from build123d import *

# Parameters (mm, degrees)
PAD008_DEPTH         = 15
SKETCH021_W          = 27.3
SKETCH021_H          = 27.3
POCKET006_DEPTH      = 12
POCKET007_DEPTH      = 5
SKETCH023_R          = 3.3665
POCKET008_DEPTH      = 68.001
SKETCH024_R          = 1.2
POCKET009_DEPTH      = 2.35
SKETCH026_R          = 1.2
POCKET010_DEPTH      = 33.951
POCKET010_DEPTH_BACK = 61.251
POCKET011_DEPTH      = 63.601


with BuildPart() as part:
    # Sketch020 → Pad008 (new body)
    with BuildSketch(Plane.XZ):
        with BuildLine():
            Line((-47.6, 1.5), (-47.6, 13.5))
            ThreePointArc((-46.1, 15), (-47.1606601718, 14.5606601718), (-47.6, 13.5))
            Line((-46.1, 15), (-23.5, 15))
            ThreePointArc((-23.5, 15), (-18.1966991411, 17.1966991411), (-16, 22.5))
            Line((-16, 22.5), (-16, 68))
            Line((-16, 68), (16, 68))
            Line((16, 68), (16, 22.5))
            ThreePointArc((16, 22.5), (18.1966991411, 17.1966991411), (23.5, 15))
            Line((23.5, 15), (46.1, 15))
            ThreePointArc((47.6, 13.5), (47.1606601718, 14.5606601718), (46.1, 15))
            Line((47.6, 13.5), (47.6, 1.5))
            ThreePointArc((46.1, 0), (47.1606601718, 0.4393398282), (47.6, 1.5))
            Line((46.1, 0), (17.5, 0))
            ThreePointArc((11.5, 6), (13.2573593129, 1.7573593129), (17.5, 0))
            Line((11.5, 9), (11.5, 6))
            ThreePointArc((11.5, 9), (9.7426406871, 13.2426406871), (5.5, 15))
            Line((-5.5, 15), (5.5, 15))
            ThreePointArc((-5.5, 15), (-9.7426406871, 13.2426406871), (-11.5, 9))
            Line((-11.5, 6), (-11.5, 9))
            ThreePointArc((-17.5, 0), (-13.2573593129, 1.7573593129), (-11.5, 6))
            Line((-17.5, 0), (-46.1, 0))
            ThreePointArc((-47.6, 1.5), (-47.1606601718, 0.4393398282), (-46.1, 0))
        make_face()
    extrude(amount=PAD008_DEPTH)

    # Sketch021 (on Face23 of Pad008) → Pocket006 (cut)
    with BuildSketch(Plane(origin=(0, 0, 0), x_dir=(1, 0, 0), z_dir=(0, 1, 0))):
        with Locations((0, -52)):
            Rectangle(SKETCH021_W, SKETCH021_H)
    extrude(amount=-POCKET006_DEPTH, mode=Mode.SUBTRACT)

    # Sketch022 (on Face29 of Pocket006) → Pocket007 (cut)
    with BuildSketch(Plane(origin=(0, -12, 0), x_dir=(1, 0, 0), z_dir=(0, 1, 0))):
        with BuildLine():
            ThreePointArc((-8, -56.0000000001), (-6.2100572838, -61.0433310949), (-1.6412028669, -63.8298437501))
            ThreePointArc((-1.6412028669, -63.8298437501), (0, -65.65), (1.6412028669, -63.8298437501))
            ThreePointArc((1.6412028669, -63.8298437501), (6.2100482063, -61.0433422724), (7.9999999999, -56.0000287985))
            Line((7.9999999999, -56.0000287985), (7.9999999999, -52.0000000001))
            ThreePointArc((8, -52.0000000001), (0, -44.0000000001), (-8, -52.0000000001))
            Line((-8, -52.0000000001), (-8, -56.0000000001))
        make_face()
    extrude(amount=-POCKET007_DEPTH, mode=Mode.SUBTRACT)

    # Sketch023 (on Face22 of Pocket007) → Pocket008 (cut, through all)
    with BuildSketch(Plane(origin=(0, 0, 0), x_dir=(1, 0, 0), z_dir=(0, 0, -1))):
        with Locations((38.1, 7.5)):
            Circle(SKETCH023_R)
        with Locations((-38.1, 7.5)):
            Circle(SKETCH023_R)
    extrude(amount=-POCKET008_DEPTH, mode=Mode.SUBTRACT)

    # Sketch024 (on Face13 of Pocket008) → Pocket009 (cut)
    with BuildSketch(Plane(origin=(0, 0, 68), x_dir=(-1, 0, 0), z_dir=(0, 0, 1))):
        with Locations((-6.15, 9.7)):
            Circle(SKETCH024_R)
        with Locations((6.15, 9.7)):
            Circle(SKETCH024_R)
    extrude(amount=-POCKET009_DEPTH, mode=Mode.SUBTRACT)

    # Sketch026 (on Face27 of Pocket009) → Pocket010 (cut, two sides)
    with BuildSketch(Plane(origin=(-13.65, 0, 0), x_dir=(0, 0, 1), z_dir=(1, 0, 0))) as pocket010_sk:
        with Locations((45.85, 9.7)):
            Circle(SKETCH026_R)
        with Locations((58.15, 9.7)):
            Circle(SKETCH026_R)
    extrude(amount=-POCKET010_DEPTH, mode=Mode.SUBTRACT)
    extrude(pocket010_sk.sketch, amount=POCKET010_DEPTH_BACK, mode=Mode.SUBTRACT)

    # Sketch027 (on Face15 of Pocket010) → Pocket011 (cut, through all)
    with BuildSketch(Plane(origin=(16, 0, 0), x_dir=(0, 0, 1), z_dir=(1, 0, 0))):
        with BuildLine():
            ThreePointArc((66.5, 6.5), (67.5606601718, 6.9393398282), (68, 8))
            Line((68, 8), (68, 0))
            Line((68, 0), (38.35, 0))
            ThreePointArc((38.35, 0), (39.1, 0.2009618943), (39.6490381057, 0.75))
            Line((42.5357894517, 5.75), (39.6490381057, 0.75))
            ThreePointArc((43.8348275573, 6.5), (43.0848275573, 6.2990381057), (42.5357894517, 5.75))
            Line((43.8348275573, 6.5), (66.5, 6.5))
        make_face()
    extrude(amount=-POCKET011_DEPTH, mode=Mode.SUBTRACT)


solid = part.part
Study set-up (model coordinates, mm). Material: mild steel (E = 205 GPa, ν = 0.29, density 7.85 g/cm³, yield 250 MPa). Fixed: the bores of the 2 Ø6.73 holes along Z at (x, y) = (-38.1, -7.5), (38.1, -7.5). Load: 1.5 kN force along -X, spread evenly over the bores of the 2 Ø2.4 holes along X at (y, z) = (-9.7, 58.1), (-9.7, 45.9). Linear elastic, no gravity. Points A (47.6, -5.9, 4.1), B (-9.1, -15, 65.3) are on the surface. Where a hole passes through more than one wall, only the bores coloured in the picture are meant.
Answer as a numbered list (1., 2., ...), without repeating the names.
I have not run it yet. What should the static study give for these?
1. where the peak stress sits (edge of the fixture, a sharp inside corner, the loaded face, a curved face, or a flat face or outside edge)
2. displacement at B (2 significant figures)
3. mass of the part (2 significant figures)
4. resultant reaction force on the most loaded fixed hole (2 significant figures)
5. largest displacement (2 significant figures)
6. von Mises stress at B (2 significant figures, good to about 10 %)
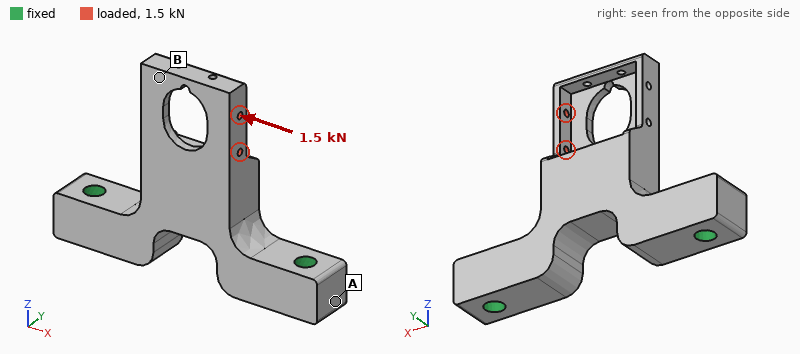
1. the loaded face
2. 40 µm
3. 230 g
4. 1.6 kN
5. 66 µm
6. 33 MPa
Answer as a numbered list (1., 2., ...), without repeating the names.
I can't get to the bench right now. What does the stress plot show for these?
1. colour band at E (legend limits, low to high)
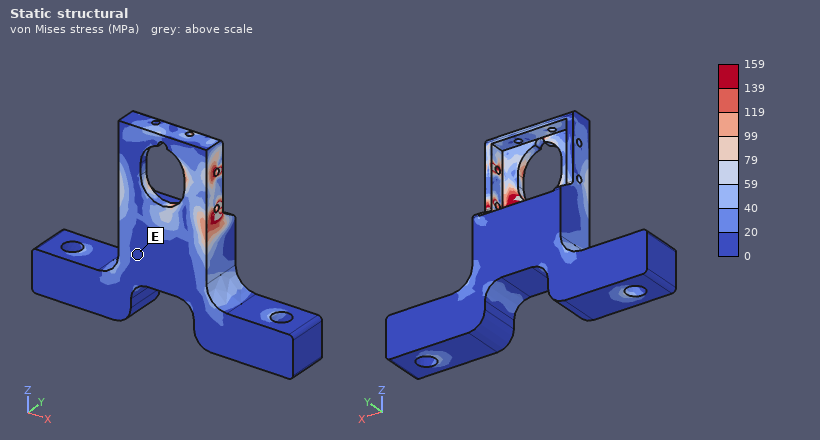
1. 0 to 20 MPa
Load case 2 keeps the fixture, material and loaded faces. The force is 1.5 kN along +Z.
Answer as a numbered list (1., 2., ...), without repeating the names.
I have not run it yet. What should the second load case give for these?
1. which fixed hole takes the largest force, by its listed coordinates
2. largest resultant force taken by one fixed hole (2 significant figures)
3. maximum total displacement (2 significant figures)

1. (38.1, -7.5)
2. 1.4 kN
3. 21 µm
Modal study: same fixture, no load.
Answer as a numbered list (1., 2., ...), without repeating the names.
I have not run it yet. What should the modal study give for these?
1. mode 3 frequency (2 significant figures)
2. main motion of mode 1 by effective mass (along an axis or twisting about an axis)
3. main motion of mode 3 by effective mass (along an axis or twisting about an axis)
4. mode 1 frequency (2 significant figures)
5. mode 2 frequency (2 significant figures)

1. 6700 Hz
2. along Y
3. along Y
4. 2700 Hz
5. 5500 Hz
